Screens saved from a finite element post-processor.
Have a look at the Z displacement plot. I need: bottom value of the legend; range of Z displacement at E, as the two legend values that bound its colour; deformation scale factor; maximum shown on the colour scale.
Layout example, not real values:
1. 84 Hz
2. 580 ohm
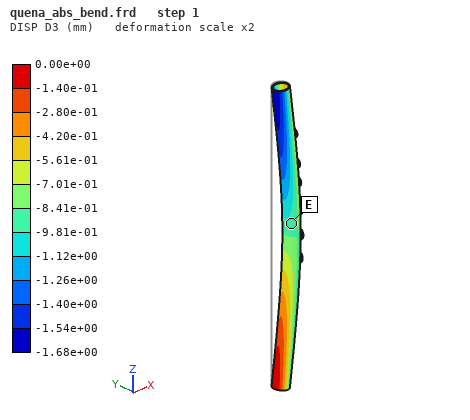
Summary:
1. -1.68e+00 mm
2. -9.81e-01 to -8.41e-01 mm
3. 2
4. 0.00e+00 mm
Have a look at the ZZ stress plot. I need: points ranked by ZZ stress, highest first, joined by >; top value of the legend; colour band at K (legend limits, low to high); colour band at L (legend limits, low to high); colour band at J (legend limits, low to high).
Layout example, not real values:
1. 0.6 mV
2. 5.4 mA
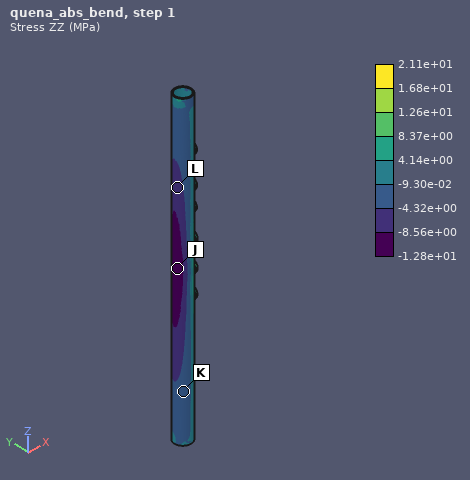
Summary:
1. K > L > J
2. 2.11e+01 MPa
3. -4.32e+00 to -9.30e-02 MPa
4. -8.56e+00 to -4.32e+00 MPa
5. -1.28e+01 to -8.56e+00 MPa
